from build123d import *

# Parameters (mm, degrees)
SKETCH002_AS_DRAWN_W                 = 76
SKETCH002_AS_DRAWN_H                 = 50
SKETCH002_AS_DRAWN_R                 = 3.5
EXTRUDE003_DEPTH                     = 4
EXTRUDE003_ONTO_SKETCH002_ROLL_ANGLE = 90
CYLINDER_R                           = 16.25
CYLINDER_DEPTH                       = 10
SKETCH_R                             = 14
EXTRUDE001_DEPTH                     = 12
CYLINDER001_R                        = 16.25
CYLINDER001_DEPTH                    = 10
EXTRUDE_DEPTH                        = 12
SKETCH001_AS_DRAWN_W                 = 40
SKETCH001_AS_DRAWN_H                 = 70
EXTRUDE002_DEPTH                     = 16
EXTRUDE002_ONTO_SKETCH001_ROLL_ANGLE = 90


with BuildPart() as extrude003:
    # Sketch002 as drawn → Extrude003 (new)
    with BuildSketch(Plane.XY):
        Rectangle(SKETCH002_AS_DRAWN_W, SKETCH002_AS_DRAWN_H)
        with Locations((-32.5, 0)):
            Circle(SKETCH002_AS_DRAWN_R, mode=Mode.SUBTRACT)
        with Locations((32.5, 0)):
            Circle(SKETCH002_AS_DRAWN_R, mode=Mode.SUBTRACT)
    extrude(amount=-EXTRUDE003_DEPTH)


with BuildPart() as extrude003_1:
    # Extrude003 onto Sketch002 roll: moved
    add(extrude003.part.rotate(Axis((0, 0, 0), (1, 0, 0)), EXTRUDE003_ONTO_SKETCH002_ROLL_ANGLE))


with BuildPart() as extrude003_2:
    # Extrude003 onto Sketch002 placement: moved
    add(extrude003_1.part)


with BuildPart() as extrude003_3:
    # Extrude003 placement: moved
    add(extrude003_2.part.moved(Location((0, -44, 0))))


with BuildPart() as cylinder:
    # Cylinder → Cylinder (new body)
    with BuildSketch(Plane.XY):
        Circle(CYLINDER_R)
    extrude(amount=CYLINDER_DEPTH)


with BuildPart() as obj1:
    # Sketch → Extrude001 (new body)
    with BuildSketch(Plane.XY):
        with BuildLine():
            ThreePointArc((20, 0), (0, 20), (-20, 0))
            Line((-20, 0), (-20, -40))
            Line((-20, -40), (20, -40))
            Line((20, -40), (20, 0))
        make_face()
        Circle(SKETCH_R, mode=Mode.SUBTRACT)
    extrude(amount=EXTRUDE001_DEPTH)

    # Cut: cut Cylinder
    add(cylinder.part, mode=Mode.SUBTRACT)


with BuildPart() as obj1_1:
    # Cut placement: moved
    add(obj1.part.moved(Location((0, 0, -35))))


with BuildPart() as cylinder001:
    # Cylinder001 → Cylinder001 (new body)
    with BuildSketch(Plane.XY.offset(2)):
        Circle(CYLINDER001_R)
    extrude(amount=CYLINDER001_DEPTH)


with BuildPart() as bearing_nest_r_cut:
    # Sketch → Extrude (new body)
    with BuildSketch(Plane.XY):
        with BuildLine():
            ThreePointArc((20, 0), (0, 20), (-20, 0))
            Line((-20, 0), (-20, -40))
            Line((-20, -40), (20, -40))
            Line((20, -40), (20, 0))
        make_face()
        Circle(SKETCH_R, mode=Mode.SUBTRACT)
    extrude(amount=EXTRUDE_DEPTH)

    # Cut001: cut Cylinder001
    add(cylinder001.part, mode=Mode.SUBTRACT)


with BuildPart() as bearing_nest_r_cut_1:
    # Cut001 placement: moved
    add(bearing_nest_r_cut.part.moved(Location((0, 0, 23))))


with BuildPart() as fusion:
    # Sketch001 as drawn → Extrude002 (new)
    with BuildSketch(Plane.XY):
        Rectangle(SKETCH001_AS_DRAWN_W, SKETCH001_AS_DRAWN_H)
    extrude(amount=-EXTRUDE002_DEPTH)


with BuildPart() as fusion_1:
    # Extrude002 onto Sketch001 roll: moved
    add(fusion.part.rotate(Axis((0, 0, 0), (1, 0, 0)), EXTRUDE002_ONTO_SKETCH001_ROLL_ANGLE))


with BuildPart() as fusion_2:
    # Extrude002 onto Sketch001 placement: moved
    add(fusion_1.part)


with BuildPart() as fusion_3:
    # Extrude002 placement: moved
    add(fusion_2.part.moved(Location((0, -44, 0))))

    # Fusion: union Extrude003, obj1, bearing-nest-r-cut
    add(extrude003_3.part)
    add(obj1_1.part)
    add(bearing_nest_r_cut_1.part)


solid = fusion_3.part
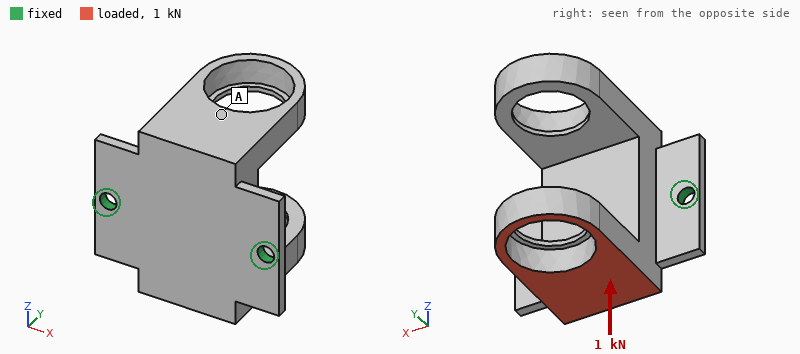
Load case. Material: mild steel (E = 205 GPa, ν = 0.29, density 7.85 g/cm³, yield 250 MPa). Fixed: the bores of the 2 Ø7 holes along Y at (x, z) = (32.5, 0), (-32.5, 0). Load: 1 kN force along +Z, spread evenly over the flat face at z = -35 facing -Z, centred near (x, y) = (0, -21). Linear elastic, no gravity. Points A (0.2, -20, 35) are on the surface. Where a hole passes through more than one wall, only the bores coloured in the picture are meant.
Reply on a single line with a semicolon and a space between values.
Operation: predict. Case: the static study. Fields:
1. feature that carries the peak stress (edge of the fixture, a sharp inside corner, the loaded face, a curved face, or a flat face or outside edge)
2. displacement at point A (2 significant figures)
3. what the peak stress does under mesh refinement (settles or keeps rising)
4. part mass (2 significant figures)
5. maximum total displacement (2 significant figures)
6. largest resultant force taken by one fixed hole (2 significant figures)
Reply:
edge of the fixture; 0.060 mm; keeps rising; 590 g; 0.12 mm; 510 N
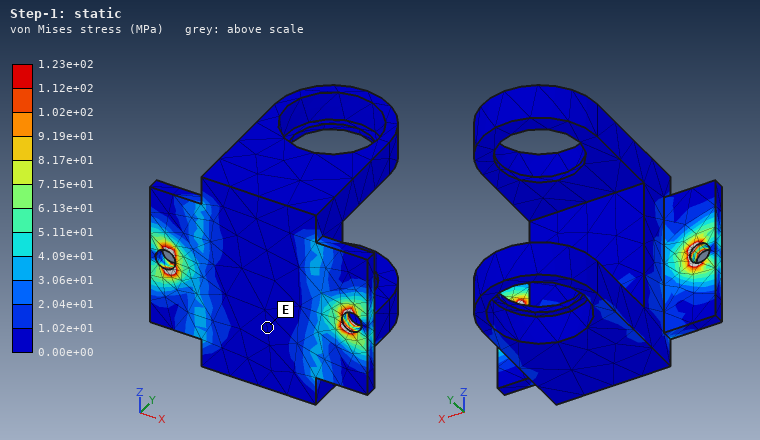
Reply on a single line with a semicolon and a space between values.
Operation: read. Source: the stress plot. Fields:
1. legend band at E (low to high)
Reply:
0.00e+00 to 1.02e+01 MPa
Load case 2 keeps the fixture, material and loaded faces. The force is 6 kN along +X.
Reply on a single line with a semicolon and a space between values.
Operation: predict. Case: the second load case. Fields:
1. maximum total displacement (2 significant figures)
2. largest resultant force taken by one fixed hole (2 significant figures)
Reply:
0.11 mm; 5.0 kN
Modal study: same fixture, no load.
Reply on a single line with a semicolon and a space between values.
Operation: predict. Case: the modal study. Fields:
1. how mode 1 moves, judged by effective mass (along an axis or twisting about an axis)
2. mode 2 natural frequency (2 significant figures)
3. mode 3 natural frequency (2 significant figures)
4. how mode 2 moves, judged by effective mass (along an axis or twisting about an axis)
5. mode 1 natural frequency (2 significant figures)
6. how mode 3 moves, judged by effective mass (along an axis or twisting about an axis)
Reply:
along Z; 2900 Hz; 3100 Hz; along Y; 810 Hz; along X
